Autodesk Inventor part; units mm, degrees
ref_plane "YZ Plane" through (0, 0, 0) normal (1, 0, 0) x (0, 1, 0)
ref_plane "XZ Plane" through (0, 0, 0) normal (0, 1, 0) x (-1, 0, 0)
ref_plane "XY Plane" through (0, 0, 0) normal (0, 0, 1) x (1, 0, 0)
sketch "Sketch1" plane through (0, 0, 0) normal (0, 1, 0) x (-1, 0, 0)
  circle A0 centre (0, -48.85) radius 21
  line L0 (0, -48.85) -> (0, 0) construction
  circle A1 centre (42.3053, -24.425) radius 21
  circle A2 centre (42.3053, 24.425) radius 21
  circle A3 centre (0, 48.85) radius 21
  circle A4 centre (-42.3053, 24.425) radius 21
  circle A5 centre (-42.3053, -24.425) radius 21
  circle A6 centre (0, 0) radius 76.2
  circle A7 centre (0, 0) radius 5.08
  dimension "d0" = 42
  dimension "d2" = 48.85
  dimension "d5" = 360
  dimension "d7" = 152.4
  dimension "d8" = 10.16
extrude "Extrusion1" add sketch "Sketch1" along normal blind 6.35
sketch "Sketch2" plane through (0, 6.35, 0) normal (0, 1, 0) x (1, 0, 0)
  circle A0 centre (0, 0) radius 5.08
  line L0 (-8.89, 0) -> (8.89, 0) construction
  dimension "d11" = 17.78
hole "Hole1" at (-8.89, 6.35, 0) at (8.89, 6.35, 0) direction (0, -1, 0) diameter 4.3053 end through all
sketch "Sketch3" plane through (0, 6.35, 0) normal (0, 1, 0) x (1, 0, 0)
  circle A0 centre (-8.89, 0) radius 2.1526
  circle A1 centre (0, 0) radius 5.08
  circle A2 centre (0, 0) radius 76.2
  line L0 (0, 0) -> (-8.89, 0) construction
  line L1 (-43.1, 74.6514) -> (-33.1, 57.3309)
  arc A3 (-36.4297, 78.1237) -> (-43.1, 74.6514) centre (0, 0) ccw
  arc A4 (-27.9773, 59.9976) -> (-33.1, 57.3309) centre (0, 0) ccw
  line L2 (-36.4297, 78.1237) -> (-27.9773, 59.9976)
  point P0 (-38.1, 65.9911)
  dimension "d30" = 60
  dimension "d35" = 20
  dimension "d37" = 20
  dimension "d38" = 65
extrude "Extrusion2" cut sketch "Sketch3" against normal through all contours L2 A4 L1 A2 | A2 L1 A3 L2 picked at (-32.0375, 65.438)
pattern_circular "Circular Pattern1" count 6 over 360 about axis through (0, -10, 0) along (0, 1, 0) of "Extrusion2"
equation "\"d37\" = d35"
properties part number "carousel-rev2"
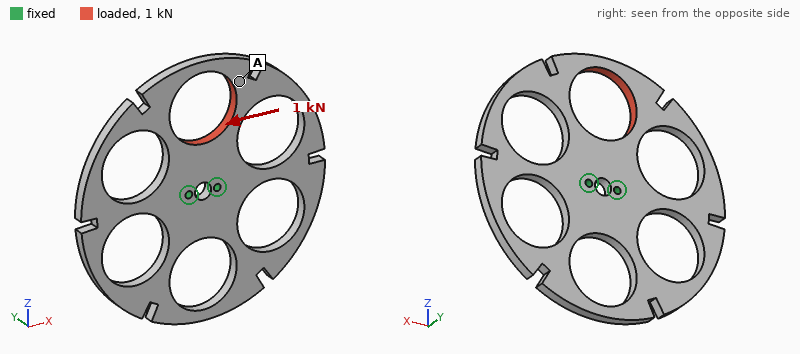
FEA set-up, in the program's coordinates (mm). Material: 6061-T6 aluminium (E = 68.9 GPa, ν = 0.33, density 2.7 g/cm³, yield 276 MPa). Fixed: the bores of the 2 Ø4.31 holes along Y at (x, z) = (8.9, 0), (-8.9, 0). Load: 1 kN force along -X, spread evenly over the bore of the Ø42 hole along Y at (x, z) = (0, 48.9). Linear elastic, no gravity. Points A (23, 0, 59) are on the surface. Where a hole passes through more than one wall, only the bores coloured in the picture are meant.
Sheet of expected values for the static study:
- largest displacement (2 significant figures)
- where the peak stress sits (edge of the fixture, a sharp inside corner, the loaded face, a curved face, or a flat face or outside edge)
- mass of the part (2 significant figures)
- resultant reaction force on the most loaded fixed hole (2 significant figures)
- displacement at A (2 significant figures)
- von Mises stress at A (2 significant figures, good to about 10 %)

80 µm
edge of the fixture
160 g
2.3 kN
64 µm
5.7 MPa
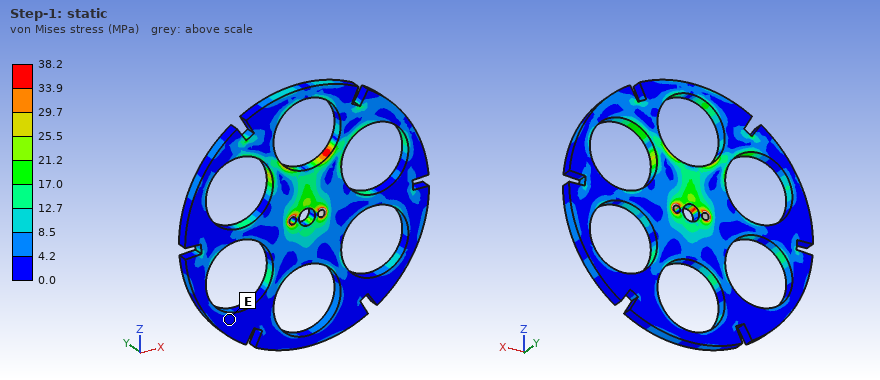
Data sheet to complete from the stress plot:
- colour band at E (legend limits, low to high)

0.0 to 4.2 MPa
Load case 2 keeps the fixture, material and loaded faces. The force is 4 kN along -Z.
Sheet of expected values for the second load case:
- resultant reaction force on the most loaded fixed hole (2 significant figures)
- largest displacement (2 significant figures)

2.0 kN
73 µm
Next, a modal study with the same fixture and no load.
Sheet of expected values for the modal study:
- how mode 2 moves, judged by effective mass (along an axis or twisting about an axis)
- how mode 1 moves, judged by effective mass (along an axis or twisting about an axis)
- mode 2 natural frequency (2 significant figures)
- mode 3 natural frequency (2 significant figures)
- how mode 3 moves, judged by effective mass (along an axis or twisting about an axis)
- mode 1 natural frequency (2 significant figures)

twisting about Z
twisting about X
820 Hz
870 Hz
along Y
710 Hz
